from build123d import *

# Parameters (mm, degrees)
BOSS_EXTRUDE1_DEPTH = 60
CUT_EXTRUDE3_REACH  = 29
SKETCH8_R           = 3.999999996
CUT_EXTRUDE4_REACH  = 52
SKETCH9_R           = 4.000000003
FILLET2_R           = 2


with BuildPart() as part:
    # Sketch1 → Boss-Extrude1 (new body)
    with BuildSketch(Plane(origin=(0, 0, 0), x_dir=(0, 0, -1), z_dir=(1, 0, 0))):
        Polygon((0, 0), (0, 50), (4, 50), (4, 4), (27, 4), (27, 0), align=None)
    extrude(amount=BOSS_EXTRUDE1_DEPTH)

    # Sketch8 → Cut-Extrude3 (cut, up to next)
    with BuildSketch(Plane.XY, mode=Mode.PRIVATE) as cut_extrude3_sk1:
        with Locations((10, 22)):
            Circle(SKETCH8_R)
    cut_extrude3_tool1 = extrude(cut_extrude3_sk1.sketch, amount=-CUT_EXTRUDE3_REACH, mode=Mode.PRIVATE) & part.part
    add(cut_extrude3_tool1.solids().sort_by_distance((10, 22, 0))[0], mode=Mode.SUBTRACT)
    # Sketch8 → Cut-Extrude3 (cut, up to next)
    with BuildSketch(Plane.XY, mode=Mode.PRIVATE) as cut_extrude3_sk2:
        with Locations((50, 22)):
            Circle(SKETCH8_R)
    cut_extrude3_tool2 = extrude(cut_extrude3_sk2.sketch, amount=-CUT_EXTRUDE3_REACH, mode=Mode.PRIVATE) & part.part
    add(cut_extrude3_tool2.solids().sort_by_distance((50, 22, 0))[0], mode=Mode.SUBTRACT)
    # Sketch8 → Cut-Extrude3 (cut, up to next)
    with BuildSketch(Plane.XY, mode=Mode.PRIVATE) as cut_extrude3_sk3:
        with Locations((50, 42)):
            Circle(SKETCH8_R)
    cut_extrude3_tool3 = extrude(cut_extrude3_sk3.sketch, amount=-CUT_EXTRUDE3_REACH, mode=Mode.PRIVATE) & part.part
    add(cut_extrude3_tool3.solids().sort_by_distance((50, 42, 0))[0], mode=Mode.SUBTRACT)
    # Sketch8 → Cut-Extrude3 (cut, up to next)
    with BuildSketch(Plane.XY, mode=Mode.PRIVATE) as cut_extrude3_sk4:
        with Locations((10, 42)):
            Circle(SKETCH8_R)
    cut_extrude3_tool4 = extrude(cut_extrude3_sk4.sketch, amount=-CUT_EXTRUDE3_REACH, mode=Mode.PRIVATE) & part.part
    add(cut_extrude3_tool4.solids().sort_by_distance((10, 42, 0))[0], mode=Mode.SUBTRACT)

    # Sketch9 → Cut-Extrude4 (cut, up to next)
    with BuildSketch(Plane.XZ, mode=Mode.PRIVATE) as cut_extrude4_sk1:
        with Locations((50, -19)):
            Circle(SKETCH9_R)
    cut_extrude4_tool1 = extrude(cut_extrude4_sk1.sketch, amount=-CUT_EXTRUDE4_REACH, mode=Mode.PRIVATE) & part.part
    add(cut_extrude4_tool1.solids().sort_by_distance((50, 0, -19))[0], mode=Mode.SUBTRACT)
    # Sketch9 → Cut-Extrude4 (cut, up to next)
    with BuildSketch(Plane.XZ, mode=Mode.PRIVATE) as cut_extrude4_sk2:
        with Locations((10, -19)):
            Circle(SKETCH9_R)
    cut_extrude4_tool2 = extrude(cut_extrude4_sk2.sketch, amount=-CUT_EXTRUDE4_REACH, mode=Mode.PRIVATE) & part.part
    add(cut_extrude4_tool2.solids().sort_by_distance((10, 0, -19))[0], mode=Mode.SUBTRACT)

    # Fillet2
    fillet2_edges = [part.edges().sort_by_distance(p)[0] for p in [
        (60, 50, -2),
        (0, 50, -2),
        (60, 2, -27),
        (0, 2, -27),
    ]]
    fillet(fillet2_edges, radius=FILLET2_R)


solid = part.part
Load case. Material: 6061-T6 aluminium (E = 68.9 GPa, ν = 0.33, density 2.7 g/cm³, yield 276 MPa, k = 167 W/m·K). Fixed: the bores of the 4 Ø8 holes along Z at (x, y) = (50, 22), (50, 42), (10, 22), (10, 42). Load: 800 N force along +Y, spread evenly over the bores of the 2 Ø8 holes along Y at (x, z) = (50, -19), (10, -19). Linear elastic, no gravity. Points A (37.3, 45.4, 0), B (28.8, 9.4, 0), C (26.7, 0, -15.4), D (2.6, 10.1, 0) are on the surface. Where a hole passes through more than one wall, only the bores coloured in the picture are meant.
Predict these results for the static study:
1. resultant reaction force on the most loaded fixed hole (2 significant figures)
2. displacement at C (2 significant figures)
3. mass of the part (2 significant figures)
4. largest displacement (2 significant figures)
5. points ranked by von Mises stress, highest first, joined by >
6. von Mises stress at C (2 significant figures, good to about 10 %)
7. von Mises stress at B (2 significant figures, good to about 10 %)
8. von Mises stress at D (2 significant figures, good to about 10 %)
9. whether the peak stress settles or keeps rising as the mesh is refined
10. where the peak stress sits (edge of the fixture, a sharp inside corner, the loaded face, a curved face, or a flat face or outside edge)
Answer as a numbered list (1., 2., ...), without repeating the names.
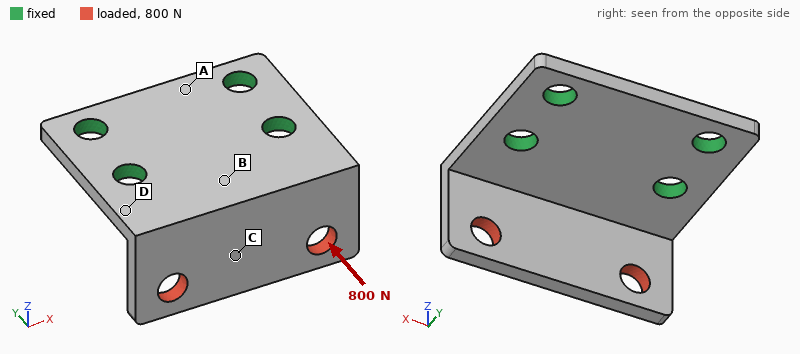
1. 340 N
2. 0.20 mm
3. 44 g
4. 0.38 mm
5. D > B > C > A
6. 25 MPa
7. 67 MPa
8. 86 MPa
9. keeps rising
10. edge of the fixture
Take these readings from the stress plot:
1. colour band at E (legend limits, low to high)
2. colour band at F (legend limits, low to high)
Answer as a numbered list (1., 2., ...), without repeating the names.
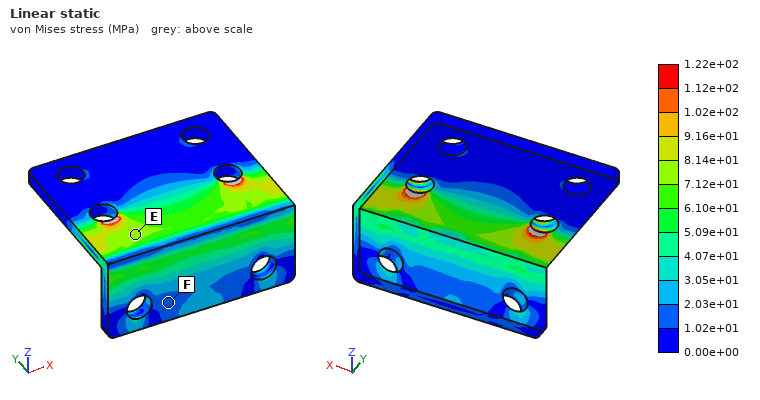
1. 7.12e+01 to 8.14e+01 MPa
2. 1.02e+01 to 2.03e+01 MPa
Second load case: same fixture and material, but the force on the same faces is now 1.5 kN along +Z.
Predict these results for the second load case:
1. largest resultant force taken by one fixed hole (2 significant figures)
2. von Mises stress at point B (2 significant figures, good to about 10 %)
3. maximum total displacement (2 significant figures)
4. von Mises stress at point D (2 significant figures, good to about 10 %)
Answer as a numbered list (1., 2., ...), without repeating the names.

1. 860 N
2. 52 MPa
3. 0.32 mm
4. 83 MPa
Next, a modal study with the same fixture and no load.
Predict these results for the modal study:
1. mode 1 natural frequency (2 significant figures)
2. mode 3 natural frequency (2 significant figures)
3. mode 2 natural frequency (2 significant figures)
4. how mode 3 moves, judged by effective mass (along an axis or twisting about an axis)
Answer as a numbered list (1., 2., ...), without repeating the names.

1. 2500 Hz
2. 6600 Hz
3. 4200 Hz
4. along Z
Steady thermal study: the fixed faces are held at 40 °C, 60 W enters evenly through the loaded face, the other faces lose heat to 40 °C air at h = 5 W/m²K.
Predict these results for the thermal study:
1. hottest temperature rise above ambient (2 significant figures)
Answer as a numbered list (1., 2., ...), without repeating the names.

1. 66 K
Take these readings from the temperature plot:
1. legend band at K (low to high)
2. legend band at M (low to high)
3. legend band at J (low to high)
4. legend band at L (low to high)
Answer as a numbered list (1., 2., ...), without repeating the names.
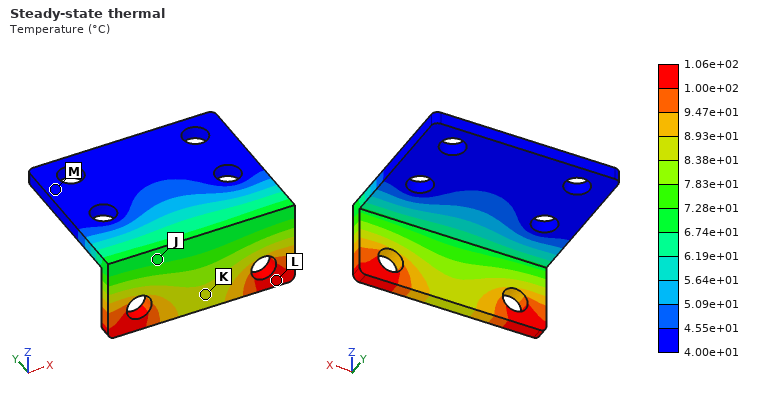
1. 8.38e+01 to 8.93e+01 °C
2. 4.00e+01 to 4.55e+01 °C
3. 6.74e+01 to 7.28e+01 °C
4. 1.00e+02 to 1.06e+02 °C
